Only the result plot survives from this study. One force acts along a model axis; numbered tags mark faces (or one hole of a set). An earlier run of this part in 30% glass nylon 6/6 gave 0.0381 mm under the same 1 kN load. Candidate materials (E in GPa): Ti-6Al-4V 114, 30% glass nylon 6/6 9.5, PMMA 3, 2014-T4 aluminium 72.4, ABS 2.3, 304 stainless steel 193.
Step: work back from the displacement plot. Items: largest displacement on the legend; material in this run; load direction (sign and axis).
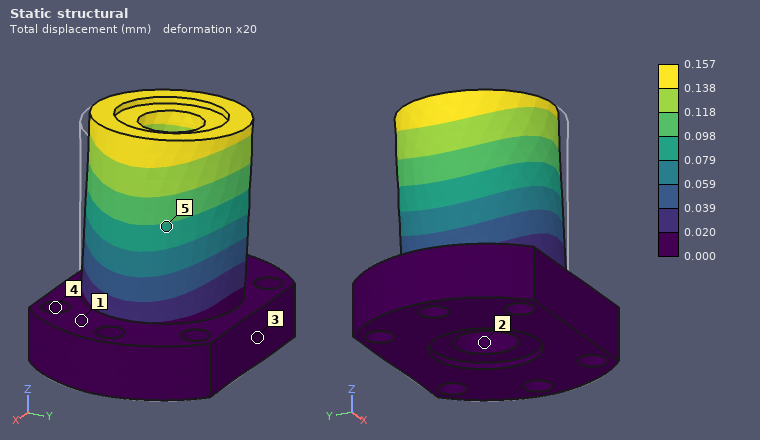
0.157 mm
ABS
-X
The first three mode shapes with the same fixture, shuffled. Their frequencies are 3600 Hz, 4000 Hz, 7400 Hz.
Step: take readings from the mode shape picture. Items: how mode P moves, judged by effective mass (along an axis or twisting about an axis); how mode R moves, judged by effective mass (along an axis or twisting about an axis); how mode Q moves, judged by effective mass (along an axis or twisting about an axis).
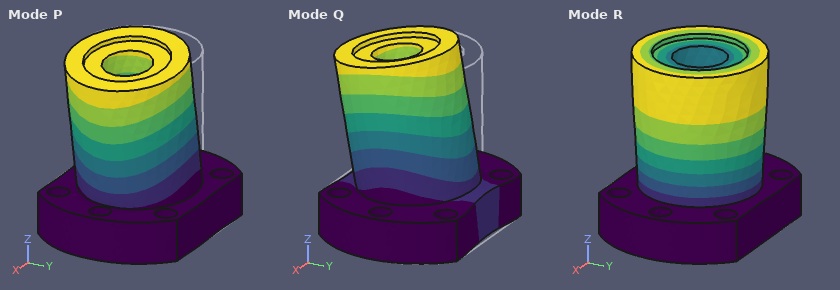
along X
twisting about Z
along Y
